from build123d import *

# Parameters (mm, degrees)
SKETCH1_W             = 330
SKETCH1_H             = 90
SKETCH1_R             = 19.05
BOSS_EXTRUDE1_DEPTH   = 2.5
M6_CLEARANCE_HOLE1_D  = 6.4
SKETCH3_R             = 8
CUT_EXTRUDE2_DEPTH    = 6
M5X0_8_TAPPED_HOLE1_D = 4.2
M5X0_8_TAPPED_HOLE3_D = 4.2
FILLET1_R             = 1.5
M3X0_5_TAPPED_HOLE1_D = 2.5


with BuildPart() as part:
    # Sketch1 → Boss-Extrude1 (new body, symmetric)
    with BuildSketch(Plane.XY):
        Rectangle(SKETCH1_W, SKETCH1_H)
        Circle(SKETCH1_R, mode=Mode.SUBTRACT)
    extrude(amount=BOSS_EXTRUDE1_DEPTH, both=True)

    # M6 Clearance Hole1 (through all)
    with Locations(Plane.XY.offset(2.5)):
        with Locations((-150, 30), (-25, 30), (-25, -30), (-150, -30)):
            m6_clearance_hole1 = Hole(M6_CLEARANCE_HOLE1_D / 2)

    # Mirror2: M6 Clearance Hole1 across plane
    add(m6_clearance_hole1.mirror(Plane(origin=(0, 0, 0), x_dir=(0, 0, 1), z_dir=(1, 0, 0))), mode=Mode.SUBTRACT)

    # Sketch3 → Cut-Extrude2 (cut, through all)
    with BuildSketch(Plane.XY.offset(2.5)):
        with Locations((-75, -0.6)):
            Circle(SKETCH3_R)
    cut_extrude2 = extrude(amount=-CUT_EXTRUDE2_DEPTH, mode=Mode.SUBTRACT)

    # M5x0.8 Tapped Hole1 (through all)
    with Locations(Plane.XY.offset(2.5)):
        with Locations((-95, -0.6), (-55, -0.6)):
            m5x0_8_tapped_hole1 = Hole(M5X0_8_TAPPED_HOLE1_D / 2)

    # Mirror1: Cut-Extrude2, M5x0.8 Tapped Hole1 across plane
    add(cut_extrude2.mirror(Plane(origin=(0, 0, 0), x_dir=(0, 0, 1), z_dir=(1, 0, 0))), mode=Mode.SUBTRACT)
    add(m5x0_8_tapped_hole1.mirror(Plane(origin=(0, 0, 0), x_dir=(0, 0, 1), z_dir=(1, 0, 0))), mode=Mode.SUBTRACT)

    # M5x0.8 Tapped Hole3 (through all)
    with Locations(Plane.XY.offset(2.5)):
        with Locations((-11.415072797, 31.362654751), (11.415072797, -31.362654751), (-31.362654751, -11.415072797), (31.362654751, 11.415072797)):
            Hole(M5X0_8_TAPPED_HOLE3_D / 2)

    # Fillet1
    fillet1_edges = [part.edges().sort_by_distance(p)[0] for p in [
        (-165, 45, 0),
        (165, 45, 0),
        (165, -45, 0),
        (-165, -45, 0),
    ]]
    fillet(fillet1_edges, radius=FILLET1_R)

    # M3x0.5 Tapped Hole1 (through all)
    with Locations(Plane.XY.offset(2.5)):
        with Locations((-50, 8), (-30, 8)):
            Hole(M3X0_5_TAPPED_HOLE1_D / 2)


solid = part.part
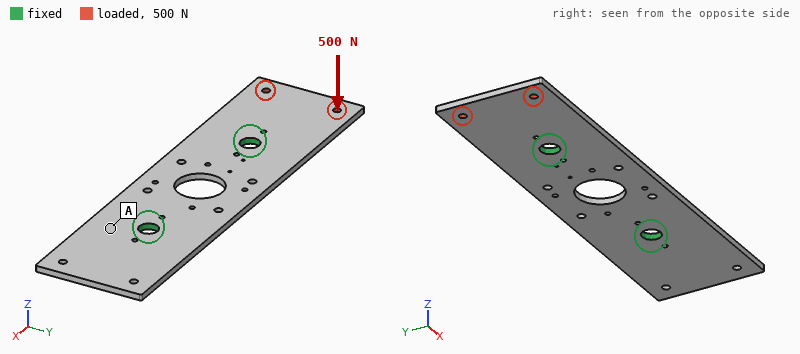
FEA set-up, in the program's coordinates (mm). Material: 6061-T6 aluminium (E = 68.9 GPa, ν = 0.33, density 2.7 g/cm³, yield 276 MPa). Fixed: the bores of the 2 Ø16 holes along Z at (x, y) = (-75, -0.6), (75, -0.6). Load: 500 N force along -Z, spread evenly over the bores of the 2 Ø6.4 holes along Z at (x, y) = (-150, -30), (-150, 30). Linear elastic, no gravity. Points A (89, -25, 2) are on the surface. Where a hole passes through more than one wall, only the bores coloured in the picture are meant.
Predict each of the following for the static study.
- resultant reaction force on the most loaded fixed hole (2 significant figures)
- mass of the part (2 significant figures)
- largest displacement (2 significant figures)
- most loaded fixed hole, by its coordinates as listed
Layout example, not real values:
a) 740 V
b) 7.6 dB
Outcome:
a) 520 N
b) 380 g
c) 1.3 mm
d) (-75, -0.6)
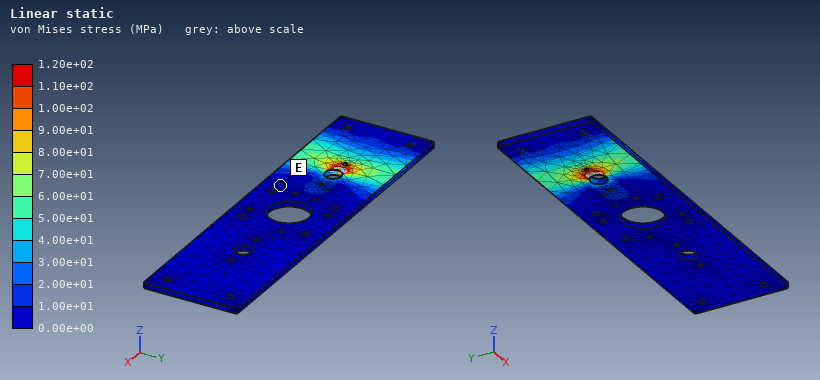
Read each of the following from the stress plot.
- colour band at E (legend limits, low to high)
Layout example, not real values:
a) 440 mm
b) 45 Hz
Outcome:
a) 0.00e+00 to 1.00e+01 MPa
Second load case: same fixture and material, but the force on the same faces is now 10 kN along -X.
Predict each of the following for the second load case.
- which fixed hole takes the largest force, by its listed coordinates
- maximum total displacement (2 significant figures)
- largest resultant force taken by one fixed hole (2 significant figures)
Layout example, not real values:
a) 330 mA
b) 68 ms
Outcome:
a) (-75, -0.6)
b) 41 µm
c) 8.9 kN
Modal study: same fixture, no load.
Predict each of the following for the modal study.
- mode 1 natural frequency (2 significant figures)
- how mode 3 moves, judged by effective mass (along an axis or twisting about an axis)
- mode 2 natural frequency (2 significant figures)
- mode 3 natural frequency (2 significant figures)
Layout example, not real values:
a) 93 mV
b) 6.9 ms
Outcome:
a) 530 Hz
b) twisting about X
c) 530 Hz
d) 1000 Hz
